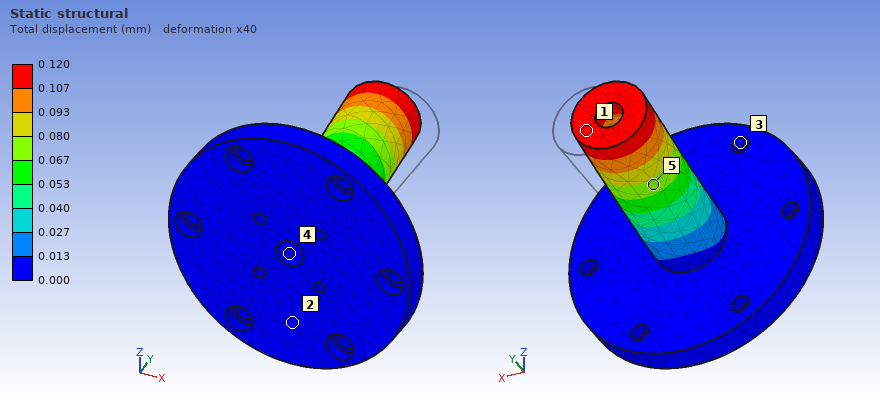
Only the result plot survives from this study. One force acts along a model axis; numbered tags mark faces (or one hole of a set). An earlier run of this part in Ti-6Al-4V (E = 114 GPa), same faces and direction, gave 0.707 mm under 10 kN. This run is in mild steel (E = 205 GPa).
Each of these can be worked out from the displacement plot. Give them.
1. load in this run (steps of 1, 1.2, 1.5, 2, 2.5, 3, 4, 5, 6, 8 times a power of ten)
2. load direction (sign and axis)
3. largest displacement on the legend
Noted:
3 kN
-X
0.120 mm
